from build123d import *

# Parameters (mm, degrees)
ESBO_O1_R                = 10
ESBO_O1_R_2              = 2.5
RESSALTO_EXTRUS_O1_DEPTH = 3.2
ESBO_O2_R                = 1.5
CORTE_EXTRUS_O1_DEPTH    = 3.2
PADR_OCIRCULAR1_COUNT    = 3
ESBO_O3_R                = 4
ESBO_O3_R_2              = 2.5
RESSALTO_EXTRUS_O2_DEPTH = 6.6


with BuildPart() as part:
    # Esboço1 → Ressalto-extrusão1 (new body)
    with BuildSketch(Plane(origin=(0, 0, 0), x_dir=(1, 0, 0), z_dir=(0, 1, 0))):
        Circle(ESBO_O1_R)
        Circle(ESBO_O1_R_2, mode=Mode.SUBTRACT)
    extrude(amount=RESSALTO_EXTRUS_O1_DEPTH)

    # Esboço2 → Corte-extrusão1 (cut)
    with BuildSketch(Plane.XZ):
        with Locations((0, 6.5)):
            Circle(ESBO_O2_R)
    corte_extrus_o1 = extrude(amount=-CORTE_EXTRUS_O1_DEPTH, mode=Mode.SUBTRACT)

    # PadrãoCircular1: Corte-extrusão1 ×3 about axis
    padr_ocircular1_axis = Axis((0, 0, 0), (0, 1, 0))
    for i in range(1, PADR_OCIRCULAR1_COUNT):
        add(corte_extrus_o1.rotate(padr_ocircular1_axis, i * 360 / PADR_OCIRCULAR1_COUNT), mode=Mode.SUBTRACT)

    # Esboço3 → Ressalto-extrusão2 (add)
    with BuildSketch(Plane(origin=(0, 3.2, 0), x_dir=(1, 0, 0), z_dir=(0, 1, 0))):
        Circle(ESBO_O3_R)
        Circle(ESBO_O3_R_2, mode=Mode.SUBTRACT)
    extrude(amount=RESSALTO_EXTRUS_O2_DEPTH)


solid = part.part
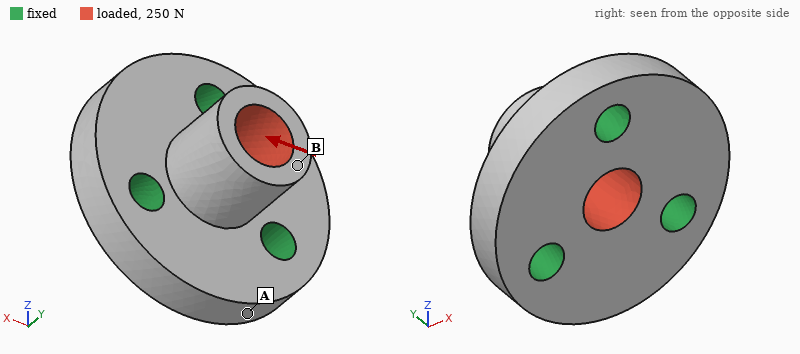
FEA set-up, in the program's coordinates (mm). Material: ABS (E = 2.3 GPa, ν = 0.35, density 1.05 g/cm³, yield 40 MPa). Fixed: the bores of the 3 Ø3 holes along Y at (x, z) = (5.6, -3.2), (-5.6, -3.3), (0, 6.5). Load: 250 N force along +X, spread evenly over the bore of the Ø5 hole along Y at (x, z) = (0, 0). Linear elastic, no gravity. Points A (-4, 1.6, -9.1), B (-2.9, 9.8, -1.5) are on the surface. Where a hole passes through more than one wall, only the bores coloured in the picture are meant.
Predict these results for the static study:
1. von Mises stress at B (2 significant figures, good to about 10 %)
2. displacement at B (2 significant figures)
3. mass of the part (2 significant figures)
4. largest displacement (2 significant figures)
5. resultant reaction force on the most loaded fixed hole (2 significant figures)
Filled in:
4.7 MPa
93 µm
1.1 g
98 µm
110 N
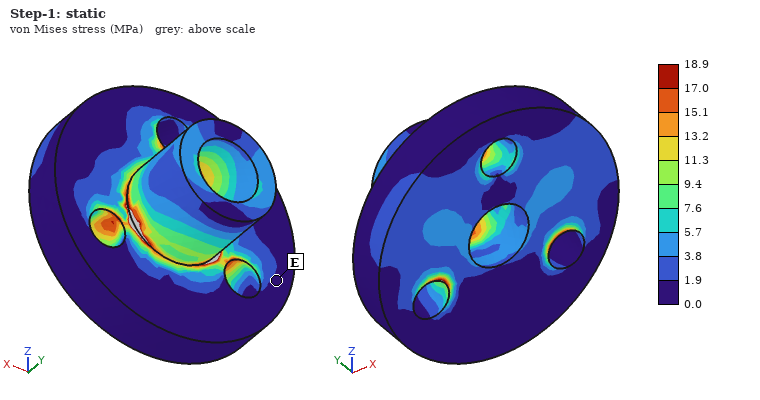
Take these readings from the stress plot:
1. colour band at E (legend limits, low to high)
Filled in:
0.0 to 1.9 MPa
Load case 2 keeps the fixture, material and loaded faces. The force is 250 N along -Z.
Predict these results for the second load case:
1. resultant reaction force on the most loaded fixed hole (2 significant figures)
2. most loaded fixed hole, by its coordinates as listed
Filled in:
120 N
(0, 6.5)
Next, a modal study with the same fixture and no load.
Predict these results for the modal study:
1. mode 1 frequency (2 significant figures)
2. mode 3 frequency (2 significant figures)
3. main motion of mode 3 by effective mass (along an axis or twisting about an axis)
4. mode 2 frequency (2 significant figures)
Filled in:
16 kHz
19 kHz
along Y
16 kHz
